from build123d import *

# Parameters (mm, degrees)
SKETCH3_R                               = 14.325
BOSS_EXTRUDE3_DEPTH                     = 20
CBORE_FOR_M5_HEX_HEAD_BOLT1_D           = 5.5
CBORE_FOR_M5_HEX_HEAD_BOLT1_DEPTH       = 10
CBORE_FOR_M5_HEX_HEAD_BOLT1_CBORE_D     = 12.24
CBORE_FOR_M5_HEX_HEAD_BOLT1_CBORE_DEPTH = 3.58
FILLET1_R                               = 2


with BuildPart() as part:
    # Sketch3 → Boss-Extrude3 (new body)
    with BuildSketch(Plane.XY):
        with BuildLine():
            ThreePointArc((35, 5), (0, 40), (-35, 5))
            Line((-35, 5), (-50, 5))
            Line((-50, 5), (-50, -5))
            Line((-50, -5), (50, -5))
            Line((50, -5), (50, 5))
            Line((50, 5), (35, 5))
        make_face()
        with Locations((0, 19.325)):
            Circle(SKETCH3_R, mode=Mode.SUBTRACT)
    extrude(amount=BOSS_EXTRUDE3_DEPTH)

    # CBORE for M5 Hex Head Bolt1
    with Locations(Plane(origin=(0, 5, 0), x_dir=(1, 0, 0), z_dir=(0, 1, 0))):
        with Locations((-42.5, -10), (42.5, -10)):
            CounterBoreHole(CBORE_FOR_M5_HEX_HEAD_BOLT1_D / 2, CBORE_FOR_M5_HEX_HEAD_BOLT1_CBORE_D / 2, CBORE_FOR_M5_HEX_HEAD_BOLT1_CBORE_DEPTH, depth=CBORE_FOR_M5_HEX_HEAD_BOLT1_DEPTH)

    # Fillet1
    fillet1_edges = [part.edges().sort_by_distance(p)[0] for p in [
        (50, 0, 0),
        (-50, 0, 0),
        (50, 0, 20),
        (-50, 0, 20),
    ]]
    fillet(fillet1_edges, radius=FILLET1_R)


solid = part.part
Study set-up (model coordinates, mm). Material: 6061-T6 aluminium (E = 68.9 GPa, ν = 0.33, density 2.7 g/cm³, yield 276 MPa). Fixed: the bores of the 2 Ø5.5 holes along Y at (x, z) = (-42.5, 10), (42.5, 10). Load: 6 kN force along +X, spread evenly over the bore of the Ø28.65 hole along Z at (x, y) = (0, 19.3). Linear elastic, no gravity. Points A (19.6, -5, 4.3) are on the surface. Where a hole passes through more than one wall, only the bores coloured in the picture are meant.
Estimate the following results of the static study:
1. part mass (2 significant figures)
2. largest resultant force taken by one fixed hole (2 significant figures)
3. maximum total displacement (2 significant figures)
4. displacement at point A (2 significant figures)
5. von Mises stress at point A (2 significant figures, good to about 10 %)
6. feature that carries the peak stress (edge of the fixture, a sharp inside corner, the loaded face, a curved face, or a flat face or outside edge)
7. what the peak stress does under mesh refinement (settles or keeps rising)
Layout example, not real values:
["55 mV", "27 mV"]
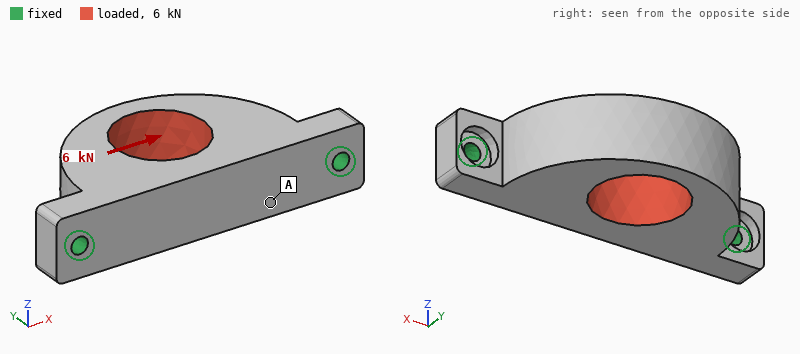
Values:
["120 g", "3.4 kN", "25 µm", "4.2 µm", "13 MPa", "edge of the fixture", "keeps rising"]
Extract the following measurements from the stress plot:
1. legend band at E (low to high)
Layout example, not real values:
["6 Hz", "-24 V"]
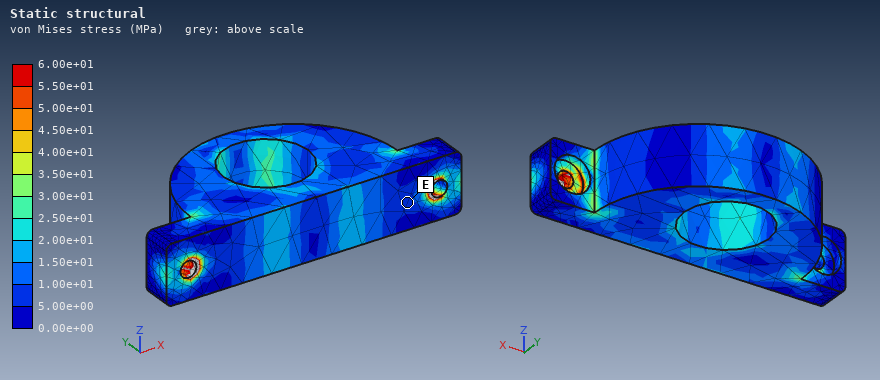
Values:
["5.00e+00 to 1.00e+01 MPa"]
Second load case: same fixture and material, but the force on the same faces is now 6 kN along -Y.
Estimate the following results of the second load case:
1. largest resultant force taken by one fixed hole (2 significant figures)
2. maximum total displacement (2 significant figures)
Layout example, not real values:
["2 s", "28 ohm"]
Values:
["3.5 kN", "33 µm"]
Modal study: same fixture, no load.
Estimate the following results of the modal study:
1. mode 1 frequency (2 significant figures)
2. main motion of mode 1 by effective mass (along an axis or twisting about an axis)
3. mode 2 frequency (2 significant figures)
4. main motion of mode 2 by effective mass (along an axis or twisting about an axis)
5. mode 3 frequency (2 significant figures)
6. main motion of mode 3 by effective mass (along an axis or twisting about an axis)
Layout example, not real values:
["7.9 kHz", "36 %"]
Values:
["2700 Hz", "along Z", "7600 Hz", "along Y", "8200 Hz", "along Z"]
